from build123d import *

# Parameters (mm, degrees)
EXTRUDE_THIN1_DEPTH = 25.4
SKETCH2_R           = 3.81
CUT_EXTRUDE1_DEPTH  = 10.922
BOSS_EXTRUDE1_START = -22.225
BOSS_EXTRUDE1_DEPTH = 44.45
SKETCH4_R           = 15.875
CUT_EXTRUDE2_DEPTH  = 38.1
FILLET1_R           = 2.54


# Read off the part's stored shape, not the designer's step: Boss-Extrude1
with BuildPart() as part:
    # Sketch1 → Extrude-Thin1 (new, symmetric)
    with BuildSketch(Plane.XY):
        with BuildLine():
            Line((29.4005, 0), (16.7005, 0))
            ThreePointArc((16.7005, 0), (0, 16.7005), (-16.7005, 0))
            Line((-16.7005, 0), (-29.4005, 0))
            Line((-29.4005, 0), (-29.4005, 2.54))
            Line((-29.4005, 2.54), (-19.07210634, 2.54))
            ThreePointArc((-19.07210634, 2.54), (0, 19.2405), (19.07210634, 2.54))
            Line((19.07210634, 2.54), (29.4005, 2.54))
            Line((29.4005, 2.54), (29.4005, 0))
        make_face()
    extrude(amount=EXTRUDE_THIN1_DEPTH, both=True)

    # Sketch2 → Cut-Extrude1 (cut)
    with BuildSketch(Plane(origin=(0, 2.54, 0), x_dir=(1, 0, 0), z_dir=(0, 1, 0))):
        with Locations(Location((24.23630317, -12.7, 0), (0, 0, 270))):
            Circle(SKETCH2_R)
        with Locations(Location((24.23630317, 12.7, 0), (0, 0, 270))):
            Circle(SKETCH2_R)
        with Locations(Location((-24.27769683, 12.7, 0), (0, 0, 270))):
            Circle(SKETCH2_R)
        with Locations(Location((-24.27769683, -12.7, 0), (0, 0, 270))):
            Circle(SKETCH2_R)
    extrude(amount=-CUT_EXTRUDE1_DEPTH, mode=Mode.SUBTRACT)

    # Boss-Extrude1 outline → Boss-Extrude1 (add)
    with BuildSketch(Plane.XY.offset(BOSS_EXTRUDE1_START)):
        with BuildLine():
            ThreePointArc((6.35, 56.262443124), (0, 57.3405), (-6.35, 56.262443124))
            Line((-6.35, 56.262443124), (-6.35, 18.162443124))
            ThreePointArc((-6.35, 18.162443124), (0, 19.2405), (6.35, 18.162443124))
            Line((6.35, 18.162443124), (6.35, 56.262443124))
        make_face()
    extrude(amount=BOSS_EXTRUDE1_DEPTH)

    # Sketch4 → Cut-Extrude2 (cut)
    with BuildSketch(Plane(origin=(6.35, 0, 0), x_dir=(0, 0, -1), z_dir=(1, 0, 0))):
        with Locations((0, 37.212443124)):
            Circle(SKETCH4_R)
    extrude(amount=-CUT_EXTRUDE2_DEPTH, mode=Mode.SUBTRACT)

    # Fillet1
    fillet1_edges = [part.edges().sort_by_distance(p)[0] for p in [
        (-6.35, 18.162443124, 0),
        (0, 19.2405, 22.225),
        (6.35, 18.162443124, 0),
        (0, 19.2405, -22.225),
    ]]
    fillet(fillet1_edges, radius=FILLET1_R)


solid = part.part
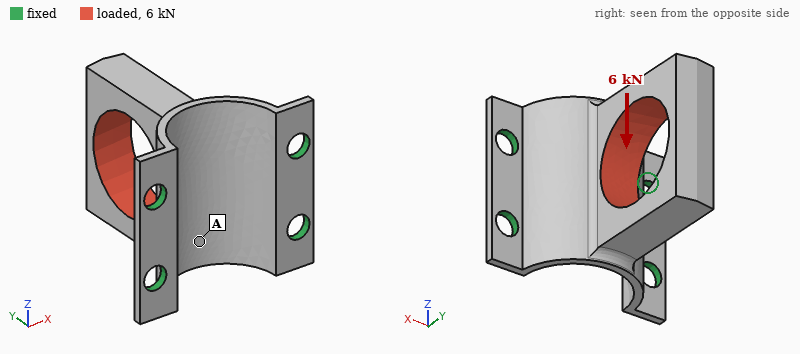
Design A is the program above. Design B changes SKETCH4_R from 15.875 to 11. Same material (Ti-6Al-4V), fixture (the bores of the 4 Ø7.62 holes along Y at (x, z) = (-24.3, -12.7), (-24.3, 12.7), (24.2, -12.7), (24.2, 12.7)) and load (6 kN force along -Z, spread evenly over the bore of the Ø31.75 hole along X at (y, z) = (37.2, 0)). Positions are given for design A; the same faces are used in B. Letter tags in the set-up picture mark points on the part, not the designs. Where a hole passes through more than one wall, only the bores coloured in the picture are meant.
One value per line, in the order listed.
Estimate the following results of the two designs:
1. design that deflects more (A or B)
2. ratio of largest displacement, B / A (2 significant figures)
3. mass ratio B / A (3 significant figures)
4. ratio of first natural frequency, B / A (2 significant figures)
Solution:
A
0.75
1.25
0.94
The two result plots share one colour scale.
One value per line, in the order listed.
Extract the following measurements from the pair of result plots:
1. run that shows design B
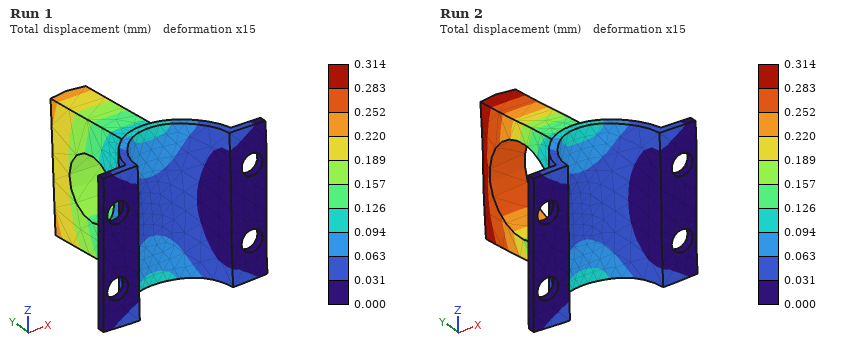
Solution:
Run 1
